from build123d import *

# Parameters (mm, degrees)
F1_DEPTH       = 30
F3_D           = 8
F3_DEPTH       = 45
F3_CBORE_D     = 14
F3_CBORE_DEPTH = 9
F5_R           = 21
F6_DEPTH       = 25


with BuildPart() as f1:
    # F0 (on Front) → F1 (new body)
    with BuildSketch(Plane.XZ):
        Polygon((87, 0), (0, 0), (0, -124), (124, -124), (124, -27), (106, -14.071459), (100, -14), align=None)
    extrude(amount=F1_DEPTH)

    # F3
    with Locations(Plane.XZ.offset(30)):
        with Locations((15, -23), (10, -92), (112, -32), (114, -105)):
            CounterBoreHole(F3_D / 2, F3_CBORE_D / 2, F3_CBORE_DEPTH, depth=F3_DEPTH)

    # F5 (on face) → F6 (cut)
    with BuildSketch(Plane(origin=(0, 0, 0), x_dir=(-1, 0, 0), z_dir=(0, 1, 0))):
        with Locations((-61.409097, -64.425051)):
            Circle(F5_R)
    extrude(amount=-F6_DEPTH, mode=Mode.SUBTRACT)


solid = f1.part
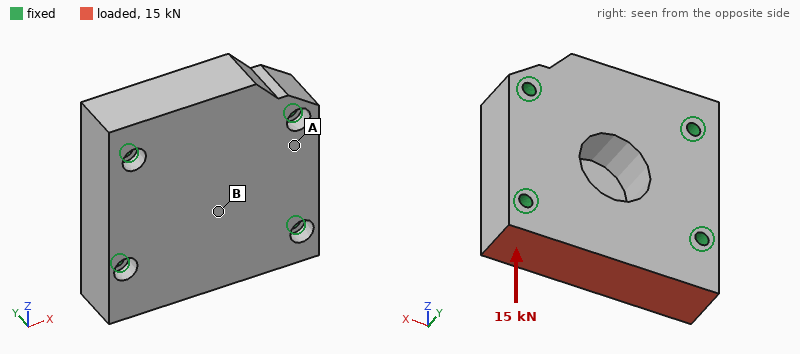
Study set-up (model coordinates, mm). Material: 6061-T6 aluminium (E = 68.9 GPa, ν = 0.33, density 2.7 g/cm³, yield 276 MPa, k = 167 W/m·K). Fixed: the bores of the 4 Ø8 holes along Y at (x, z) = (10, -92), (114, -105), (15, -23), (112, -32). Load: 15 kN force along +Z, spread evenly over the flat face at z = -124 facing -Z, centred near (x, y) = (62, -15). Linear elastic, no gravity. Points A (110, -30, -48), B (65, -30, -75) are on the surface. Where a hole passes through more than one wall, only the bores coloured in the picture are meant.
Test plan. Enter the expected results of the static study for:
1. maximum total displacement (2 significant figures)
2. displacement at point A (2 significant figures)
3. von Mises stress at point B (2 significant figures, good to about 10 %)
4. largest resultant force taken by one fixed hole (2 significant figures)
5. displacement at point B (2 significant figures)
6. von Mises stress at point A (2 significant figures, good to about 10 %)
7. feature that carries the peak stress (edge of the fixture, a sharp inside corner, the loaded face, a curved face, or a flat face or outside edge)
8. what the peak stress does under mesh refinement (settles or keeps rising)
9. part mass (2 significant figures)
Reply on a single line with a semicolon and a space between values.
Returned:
6.7 µm; 1.4 µm; 5.6 MPa; 5.4 kN; 3.8 µm; 2.4 MPa; edge of the fixture; keeps rising; 1.1 kg
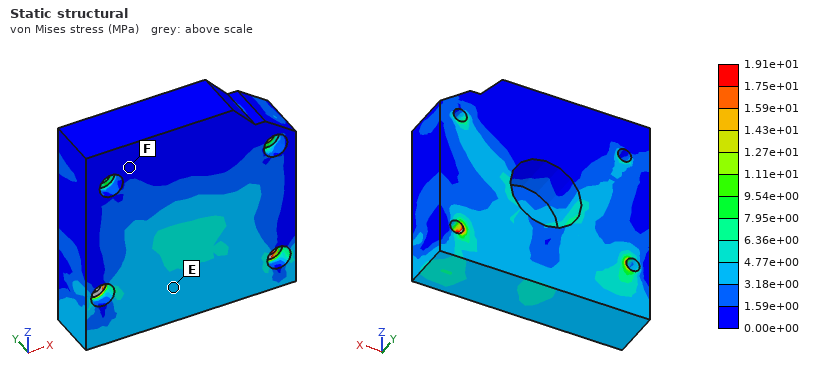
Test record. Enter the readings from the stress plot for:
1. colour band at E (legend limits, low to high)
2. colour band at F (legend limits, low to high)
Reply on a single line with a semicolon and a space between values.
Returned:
3.18e+00 to 4.77e+00 MPa; 0.00e+00 to 1.59e+00 MPa
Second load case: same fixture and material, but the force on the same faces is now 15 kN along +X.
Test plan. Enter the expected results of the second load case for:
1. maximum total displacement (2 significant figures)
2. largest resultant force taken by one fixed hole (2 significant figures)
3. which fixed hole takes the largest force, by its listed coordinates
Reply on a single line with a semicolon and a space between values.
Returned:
12 µm; 8.4 kN; (114, -105)
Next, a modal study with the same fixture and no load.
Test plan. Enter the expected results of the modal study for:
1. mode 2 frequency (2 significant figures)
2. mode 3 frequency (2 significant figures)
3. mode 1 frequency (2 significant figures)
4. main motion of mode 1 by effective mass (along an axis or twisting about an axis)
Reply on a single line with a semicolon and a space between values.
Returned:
8200 Hz; 11 kHz; 7300 Hz; along Y
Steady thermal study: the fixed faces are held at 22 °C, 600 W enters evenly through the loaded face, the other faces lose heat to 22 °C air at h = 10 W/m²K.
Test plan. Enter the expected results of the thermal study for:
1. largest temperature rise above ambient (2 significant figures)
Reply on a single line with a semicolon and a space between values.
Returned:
52 K
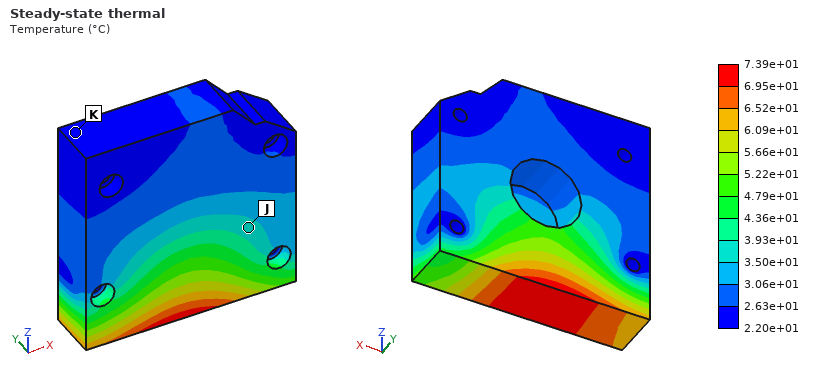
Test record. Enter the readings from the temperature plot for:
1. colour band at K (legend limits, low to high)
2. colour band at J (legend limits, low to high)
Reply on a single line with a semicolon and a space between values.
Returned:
2.20e+01 to 2.63e+01 °C; 3.50e+01 to 3.93e+01 °C
